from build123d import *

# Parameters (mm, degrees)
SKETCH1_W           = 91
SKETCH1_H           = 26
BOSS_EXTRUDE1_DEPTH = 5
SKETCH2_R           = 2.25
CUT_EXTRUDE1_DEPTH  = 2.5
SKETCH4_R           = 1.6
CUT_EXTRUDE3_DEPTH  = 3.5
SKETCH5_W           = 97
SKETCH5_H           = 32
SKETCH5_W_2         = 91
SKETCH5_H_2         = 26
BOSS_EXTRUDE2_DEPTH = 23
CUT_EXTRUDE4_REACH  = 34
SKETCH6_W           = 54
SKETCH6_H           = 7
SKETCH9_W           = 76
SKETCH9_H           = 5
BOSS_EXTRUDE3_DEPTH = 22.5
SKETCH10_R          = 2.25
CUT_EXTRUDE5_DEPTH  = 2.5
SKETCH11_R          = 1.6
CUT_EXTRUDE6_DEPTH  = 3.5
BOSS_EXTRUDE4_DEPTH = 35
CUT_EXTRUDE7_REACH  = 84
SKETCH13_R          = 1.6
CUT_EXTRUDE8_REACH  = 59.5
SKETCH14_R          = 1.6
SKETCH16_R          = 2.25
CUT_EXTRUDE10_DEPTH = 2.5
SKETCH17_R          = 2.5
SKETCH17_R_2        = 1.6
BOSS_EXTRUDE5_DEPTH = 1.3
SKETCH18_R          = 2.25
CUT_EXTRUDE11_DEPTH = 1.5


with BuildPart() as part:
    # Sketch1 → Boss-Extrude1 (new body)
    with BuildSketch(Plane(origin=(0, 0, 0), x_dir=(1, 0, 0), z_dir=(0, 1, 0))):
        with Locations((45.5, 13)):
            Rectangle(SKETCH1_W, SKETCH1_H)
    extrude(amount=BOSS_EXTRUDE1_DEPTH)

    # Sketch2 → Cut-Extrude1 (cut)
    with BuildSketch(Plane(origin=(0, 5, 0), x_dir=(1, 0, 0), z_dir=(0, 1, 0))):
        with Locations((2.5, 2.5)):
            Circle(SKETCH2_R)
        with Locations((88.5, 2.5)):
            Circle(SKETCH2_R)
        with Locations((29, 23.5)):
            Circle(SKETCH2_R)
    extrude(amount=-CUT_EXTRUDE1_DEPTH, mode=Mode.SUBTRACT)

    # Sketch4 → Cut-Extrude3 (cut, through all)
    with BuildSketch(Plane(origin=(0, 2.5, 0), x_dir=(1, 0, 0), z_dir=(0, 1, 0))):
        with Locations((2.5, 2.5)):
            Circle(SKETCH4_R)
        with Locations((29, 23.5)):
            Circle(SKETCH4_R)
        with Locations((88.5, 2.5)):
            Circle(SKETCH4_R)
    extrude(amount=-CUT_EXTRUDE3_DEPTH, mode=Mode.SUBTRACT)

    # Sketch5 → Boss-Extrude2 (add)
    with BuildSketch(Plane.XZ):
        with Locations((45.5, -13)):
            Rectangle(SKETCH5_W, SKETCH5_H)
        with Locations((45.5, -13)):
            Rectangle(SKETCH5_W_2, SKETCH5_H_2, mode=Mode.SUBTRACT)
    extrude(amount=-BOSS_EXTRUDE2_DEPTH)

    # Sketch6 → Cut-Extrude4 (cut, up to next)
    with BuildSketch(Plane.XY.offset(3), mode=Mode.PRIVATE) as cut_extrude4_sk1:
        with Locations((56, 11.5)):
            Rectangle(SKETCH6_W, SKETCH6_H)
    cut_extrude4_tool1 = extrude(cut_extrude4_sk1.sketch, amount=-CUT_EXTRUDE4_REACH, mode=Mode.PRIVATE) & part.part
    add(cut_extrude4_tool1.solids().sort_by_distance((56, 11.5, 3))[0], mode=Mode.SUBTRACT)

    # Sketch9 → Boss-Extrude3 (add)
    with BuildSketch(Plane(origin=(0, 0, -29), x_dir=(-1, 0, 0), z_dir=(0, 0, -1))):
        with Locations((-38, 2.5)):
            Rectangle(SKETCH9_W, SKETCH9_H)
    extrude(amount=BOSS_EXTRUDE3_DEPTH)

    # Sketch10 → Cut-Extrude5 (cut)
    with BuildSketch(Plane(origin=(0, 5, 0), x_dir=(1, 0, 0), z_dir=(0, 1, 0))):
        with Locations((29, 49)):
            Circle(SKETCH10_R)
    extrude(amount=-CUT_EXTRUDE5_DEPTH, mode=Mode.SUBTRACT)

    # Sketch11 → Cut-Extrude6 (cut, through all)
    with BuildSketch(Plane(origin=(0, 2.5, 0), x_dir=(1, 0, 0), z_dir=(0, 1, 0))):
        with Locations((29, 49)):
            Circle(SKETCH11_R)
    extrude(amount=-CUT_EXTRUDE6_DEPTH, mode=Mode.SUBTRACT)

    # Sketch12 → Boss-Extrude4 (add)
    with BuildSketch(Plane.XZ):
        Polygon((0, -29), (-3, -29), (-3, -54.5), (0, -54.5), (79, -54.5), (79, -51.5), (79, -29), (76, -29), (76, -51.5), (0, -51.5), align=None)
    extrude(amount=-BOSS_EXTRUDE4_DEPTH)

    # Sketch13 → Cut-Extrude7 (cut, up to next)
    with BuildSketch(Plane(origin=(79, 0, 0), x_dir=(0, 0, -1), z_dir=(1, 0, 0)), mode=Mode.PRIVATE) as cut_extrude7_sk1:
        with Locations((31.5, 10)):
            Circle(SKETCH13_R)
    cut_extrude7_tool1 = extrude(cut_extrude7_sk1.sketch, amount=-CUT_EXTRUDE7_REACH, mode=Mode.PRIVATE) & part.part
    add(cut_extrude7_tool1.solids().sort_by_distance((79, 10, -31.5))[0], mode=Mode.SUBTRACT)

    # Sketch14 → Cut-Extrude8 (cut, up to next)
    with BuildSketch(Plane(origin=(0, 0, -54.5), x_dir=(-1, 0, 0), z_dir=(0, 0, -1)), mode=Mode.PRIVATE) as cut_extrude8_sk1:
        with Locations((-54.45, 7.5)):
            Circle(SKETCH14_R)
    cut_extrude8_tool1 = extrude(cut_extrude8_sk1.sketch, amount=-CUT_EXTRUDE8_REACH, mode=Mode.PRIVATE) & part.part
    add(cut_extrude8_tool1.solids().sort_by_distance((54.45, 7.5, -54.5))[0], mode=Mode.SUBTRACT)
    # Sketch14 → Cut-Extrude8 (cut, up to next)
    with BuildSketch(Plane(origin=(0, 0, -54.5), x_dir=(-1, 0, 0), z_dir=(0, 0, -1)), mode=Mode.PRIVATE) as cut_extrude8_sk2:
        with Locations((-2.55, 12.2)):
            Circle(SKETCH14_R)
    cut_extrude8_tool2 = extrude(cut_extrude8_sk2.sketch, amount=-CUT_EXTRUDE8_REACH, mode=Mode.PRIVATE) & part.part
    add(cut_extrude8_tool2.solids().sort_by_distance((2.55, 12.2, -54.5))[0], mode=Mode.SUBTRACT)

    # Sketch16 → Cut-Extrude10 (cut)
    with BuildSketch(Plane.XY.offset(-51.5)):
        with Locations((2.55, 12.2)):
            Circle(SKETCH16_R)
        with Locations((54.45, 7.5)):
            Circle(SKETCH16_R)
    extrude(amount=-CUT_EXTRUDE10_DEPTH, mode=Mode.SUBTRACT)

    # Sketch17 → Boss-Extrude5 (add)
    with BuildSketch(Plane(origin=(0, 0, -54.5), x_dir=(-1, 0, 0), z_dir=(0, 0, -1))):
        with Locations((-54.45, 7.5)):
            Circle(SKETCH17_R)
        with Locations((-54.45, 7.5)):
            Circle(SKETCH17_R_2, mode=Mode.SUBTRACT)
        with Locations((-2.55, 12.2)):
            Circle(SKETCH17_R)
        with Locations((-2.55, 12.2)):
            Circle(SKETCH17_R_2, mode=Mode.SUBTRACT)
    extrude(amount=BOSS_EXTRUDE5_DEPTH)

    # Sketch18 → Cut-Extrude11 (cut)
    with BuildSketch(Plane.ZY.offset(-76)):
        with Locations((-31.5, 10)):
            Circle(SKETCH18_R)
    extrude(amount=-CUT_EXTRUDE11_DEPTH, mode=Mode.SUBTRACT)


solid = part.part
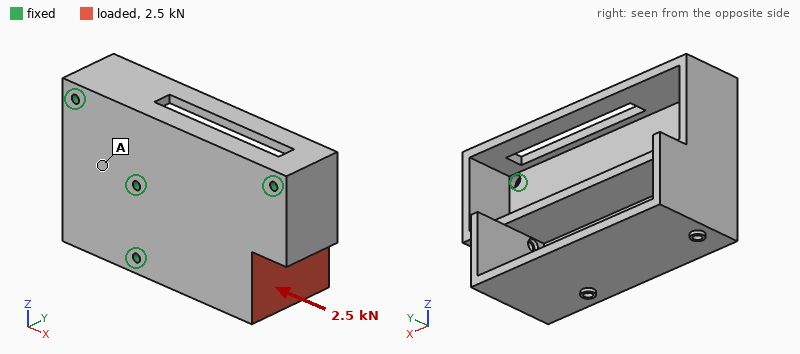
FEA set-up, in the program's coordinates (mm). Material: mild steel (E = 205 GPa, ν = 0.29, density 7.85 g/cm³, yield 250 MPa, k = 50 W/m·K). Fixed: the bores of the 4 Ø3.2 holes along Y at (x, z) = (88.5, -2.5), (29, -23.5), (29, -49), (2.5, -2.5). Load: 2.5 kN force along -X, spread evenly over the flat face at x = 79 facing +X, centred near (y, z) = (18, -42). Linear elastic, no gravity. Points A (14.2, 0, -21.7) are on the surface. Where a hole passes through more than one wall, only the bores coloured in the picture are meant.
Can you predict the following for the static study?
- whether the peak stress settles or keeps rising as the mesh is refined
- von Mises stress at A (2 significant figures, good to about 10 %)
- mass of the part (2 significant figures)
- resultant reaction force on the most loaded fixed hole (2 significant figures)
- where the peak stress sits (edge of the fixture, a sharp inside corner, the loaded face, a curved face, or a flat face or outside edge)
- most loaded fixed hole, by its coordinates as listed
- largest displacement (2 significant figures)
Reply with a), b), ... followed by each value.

a) keeps rising
b) 16 MPa
c) 390 g
d) 1.1 kN
e) edge of the fixture
f) (88.5, -2.5)
g) 0.11 mm
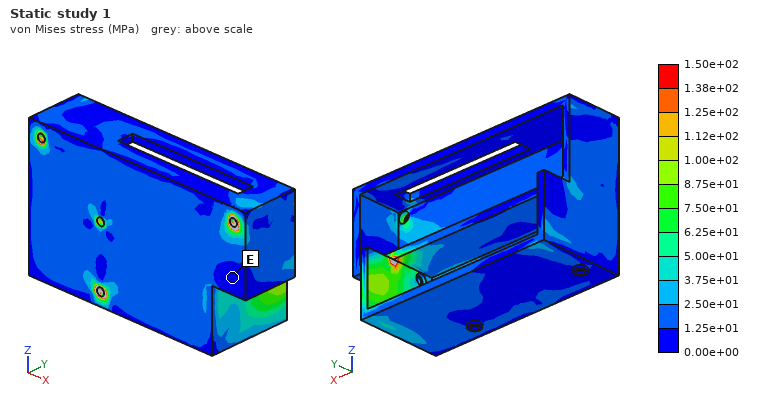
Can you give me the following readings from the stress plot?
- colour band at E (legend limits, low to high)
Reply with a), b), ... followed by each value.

a) 0.00e+00 to 1.25e+01 MPa
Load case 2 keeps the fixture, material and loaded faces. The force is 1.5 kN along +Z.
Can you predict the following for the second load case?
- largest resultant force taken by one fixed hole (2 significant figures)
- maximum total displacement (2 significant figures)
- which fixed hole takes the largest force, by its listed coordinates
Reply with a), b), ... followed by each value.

a) 1.1 kN
b) 0.10 mm
c) (29, -49)
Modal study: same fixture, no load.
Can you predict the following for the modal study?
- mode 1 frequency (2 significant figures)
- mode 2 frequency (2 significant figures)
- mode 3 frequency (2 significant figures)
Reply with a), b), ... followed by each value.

a) 1700 Hz
b) 3000 Hz
c) 3600 Hz
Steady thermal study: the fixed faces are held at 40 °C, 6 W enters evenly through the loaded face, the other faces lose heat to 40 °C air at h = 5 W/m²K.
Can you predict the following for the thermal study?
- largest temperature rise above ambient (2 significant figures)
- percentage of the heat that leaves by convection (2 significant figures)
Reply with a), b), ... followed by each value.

a) 21 K
b) 11 %
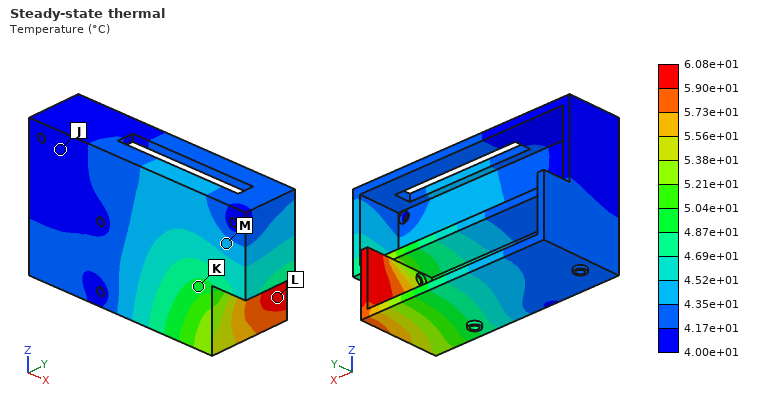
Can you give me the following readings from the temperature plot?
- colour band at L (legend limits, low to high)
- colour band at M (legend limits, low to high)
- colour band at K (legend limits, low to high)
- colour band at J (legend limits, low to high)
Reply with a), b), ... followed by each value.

a) 5.90e+01 to 6.08e+01 °C
b) 4.35e+01 to 4.52e+01 °C
c) 4.87e+01 to 5.04e+01 °C
d) 4.00e+01 to 4.17e+01 °C
